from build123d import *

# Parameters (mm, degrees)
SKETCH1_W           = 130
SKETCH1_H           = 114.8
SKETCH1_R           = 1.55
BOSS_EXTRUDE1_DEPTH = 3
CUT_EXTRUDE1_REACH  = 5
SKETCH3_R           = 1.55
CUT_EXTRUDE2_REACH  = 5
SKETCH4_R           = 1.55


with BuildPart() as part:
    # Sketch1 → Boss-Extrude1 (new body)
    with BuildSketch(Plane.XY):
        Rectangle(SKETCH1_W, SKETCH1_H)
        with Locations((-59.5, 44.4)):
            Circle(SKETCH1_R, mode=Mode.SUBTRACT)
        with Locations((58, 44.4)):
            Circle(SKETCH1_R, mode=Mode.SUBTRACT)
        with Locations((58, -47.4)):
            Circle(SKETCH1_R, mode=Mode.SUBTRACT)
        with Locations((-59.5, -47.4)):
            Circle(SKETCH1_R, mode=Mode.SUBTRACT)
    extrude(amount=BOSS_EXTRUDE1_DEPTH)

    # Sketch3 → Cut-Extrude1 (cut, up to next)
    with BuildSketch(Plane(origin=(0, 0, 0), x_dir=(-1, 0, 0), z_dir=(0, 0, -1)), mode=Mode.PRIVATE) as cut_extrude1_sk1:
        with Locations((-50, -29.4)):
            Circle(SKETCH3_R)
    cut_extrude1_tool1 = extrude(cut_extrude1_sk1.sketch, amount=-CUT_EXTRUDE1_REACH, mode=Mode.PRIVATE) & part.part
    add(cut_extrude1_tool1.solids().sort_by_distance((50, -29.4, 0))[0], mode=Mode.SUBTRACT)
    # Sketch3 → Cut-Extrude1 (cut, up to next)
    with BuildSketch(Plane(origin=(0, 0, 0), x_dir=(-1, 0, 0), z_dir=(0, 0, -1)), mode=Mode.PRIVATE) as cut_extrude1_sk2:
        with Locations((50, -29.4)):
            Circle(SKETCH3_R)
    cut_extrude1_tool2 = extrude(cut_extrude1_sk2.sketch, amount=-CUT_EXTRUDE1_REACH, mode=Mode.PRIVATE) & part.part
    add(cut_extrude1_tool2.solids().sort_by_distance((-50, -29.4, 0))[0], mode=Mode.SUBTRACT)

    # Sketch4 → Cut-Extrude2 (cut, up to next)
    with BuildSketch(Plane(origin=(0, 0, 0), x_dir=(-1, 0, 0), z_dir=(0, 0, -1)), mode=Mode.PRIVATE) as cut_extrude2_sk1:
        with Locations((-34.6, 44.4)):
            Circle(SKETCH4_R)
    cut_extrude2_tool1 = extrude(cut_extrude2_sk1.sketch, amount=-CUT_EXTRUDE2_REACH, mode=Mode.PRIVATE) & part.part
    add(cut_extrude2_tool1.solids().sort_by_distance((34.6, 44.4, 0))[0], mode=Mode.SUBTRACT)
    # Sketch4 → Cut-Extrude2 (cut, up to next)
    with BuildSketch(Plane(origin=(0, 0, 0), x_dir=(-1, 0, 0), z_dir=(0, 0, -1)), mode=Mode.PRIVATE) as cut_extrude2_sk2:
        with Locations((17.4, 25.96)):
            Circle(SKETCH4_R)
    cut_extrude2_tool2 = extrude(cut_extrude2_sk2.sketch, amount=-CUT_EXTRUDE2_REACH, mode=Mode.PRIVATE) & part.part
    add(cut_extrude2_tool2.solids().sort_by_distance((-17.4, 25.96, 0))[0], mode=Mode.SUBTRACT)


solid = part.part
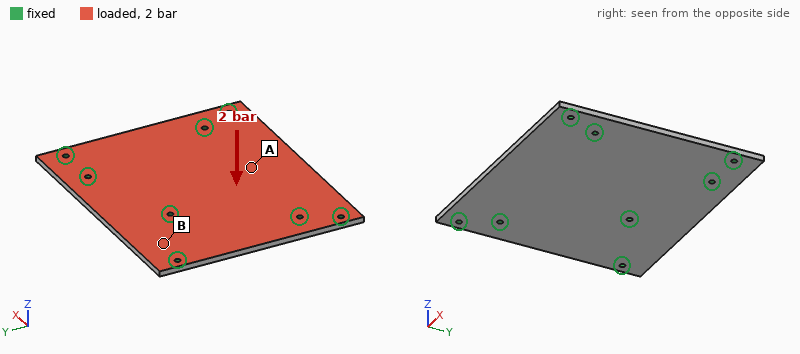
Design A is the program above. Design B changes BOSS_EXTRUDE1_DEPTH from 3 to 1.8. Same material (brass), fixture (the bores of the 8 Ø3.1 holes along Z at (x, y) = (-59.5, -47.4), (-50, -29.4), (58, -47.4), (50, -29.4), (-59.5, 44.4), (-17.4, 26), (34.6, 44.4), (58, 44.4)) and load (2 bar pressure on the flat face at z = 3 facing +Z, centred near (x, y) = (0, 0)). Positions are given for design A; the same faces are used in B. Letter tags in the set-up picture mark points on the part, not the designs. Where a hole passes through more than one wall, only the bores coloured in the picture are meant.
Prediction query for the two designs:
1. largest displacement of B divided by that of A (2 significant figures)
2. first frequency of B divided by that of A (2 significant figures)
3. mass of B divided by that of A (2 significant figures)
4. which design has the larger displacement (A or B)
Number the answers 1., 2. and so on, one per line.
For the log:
1. 4.5
2. 0.61
3. 0.60
4. B
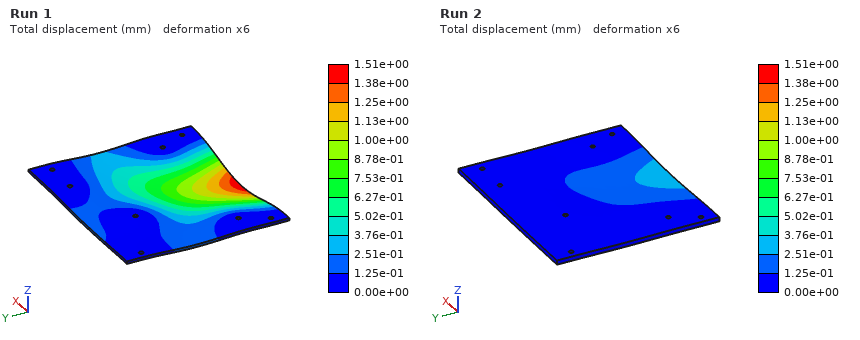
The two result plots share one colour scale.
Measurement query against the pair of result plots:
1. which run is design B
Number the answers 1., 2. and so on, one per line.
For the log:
1. Run 1
